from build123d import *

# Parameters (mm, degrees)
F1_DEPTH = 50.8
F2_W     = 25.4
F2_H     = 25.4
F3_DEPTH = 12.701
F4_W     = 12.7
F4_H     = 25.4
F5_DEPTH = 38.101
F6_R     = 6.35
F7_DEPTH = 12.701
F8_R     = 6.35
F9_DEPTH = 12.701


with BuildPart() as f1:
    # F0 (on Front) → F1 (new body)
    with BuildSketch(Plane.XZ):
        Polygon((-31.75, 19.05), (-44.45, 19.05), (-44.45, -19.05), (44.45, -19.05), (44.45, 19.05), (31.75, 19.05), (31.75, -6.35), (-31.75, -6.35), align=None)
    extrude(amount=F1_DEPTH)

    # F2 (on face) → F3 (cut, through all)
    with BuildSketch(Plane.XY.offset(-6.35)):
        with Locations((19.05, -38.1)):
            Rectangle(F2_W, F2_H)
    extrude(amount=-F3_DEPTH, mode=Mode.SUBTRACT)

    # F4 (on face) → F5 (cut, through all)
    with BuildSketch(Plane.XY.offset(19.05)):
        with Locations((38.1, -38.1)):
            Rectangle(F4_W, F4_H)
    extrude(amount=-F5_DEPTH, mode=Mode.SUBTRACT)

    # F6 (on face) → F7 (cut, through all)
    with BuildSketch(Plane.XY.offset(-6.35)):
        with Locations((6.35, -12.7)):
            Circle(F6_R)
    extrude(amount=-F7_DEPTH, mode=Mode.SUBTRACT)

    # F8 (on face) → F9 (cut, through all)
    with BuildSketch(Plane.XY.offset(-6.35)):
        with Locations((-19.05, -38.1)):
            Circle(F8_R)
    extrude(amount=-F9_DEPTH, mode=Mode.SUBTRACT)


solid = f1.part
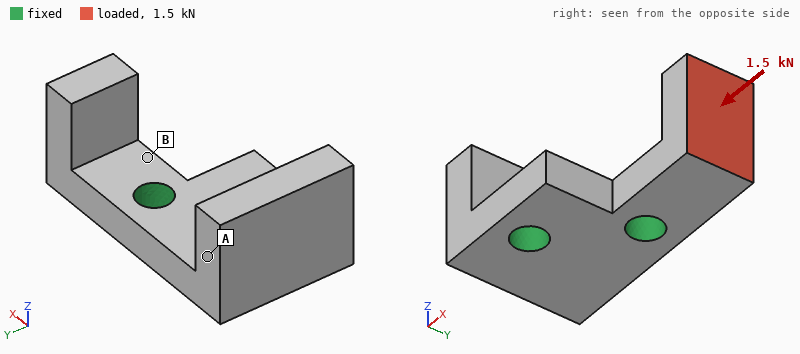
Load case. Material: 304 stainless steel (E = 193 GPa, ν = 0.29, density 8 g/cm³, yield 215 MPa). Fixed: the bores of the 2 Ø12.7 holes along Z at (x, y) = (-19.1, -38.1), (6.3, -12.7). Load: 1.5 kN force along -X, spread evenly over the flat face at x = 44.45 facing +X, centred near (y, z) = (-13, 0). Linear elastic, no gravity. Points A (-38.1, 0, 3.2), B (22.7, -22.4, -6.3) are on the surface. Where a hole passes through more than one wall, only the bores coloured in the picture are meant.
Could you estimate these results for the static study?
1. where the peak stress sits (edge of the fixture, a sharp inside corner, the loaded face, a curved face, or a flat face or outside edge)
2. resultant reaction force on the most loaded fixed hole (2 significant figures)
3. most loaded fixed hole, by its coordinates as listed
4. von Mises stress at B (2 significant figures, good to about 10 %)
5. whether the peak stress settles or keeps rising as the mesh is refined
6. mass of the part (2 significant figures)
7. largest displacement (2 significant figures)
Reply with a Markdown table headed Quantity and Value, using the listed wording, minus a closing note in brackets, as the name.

| Quantity | Value |
|---|---|
| where the peak stress sits | edge of the fixture |
| resultant reaction force on the most loaded fixed hole | 1.5 kN |
| most loaded fixed hole, by its coordinates as listed | (6.3, -12.7) |
| von Mises stress at B | 30 MPa |
| whether the peak stress settles or keeps rising as the mesh is refined | keeps rising |
| mass of the part | 530 g |
| largest displacement | 27 µm |
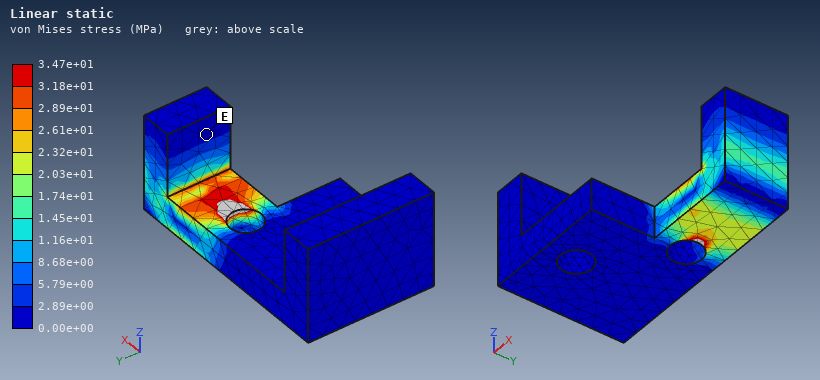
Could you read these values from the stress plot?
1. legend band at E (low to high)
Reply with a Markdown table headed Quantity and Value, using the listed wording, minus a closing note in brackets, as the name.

| Quantity | Value |
|---|---|
| legend band at E | 0.00e+00 to 2.89e+00 MPa |
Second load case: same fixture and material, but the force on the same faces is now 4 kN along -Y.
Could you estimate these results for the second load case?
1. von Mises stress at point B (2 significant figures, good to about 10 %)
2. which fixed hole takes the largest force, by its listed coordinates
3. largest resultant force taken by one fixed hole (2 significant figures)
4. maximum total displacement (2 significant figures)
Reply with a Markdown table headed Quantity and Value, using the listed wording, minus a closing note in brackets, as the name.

| Quantity | Value |
|---|---|
| von Mises stress at point B | 75 MPa |
| which fixed hole takes the largest force, by its listed coordinates | (6.3, -12.7) |
| largest resultant force taken by one fixed hole | 4.5 kN |
| maximum total displacement | 73 µm |
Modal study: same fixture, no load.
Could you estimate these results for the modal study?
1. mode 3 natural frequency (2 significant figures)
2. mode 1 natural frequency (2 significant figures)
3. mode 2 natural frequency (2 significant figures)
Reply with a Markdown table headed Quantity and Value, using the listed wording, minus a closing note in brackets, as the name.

| Quantity | Value |
|---|---|
| mode 3 natural frequency | 4700 Hz |
| mode 1 natural frequency | 3700 Hz |
| mode 2 natural frequency | 4500 Hz |
